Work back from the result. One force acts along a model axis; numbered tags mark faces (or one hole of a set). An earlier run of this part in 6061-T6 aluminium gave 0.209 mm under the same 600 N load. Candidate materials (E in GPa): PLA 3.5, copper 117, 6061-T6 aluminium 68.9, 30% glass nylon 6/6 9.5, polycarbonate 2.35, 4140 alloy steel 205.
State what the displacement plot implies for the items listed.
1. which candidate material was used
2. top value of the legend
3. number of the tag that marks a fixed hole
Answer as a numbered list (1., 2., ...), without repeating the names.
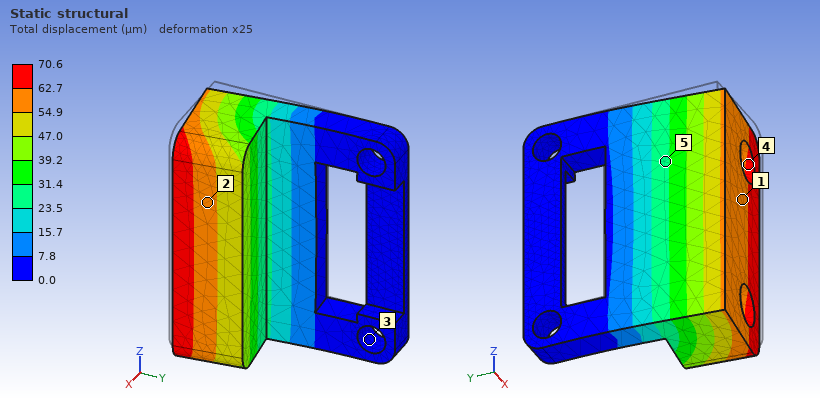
1. 4140 alloy steel
2. 70.6 µm
3. 3
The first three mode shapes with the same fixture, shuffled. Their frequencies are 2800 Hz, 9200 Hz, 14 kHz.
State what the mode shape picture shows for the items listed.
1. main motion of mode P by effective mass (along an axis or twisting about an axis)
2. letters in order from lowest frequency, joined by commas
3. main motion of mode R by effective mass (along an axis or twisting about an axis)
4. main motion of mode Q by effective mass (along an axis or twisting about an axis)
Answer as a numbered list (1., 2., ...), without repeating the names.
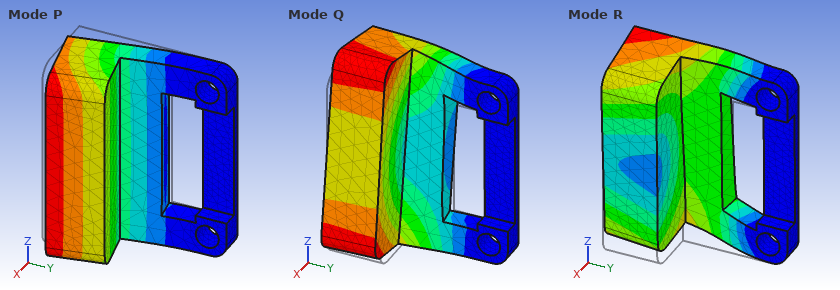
1. along X
2. P, Q, R
3. along Z
4. along Z
